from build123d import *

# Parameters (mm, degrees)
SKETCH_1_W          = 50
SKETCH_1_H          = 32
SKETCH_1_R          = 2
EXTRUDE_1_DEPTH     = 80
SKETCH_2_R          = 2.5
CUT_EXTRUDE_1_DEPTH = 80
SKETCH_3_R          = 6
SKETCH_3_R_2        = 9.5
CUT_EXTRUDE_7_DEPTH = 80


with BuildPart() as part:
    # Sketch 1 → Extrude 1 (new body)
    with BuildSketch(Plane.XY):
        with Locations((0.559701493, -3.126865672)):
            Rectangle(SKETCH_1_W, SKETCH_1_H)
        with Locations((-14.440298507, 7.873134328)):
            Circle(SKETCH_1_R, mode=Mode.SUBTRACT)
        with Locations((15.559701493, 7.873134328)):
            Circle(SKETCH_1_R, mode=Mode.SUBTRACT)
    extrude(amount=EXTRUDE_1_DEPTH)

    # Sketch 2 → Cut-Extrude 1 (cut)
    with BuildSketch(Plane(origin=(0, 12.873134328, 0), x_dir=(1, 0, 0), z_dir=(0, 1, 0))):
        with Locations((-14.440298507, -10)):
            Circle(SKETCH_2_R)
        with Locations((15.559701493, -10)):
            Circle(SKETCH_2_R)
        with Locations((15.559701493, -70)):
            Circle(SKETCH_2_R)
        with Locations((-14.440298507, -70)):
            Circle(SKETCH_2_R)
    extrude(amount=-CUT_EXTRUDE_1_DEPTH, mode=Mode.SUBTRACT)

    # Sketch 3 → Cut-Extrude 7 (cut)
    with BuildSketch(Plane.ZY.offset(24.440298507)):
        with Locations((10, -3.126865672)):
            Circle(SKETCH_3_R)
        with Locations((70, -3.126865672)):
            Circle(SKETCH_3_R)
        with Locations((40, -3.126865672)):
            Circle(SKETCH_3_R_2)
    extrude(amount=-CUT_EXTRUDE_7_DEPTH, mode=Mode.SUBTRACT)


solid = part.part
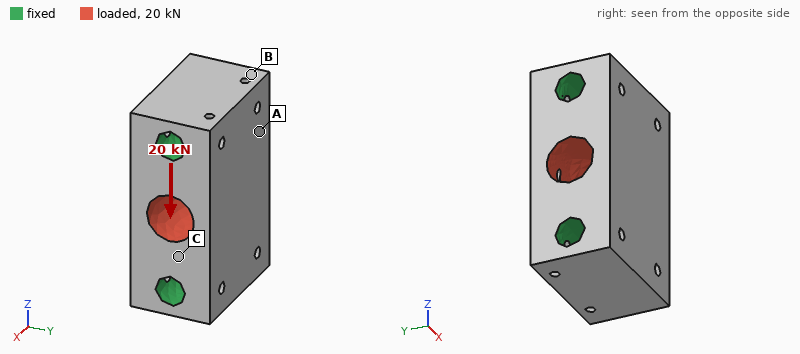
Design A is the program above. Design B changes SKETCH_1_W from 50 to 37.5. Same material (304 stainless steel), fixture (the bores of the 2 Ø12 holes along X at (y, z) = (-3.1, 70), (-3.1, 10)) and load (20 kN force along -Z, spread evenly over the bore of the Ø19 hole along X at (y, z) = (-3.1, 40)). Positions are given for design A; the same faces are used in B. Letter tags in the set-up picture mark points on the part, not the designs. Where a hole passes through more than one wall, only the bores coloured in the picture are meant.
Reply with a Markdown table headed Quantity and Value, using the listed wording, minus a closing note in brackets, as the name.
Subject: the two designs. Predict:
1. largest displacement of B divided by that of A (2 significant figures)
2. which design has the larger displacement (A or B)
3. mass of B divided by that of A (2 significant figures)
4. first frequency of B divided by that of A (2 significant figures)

| Quantity | Value |
|---|---|
| largest displacement of B divided by that of A | 1.4 |
| which design has the larger displacement | B |
| mass of B divided by that of A | 0.74 |
| first frequency of B divided by that of A | 1.00 |
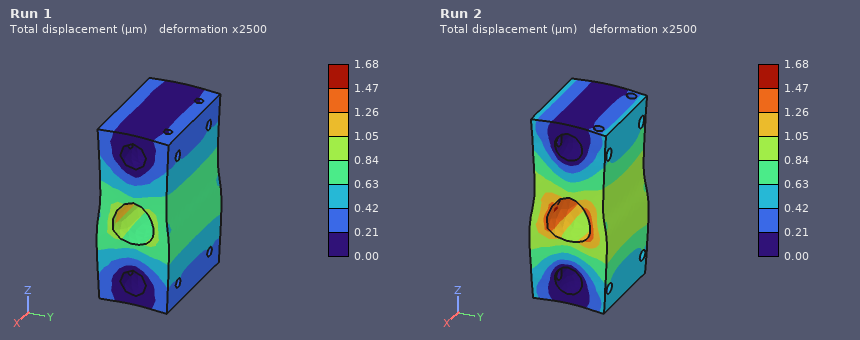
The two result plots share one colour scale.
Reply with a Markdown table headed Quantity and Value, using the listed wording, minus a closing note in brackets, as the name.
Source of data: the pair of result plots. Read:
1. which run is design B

| Quantity | Value |
|---|---|
| which run is design B | Run 2 |
